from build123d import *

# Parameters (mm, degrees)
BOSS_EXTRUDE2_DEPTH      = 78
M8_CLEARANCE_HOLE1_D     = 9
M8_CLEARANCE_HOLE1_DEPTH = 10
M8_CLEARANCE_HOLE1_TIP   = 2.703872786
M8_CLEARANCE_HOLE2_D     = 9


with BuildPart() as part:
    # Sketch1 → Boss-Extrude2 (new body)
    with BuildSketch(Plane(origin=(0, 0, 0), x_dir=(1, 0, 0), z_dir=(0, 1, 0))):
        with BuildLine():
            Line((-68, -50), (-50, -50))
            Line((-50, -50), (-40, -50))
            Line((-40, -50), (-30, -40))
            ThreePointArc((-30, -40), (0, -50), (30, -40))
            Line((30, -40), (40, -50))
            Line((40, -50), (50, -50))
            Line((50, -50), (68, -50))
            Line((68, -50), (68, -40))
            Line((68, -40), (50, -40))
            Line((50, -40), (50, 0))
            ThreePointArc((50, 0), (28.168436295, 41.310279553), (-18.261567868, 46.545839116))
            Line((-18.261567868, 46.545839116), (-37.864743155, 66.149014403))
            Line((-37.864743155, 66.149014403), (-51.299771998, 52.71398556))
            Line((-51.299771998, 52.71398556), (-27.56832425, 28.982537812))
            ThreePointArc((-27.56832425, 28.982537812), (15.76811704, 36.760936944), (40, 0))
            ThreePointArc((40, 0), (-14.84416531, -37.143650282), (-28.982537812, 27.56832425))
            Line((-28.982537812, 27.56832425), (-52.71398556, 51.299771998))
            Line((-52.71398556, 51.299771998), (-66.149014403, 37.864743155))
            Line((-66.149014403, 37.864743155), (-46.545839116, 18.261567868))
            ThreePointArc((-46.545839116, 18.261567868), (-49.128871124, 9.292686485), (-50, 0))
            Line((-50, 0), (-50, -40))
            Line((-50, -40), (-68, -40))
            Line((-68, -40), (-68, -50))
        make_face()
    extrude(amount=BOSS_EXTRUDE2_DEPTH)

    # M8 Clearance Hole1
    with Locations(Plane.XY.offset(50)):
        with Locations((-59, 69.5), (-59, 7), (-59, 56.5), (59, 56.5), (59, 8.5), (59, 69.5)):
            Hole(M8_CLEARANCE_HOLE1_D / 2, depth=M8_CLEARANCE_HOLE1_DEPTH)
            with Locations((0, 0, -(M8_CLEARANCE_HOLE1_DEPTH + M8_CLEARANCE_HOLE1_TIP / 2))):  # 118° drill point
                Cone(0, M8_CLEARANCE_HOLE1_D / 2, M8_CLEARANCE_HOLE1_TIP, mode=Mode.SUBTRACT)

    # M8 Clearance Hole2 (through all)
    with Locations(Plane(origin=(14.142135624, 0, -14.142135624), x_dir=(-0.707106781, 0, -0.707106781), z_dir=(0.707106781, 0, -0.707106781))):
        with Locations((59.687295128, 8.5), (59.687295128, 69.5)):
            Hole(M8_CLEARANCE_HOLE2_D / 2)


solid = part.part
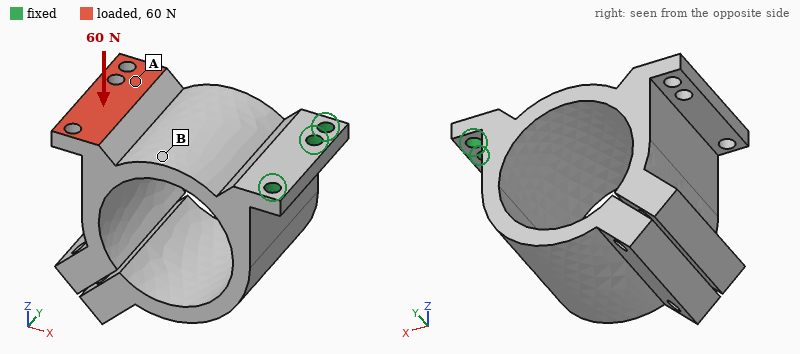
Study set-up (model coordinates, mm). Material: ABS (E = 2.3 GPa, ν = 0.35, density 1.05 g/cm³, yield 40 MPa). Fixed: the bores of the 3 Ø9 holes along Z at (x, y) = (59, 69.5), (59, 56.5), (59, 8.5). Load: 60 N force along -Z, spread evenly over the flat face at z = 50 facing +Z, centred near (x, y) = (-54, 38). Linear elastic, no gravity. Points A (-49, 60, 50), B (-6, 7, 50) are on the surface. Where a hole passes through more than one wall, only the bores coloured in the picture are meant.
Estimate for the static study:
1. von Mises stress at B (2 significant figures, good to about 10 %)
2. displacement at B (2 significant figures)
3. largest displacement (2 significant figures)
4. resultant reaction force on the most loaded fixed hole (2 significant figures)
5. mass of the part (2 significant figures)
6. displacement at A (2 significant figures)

2.0 MPa
0.55 mm
2.3 mm
30 N
390 g
1.3 mm
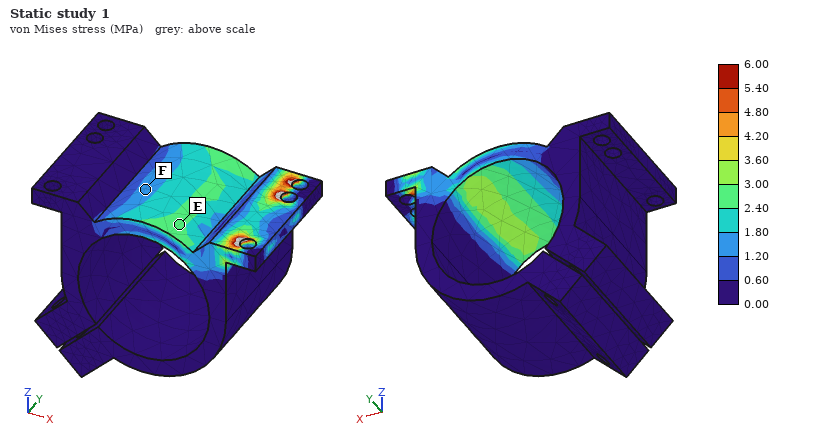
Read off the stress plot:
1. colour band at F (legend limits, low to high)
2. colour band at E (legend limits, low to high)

1.20 to 1.80 MPa
2.40 to 3.00 MPa
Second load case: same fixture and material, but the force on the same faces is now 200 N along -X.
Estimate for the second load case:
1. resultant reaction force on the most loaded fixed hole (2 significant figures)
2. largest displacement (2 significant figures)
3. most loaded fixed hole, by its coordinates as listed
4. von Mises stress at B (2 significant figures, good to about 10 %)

90 N
0.93 mm
(59, 8.5)
1.00 MPa
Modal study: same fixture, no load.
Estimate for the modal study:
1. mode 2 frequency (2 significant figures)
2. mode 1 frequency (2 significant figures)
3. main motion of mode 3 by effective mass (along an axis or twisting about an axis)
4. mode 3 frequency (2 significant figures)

110 Hz
70 Hz
along Y
170 Hz
